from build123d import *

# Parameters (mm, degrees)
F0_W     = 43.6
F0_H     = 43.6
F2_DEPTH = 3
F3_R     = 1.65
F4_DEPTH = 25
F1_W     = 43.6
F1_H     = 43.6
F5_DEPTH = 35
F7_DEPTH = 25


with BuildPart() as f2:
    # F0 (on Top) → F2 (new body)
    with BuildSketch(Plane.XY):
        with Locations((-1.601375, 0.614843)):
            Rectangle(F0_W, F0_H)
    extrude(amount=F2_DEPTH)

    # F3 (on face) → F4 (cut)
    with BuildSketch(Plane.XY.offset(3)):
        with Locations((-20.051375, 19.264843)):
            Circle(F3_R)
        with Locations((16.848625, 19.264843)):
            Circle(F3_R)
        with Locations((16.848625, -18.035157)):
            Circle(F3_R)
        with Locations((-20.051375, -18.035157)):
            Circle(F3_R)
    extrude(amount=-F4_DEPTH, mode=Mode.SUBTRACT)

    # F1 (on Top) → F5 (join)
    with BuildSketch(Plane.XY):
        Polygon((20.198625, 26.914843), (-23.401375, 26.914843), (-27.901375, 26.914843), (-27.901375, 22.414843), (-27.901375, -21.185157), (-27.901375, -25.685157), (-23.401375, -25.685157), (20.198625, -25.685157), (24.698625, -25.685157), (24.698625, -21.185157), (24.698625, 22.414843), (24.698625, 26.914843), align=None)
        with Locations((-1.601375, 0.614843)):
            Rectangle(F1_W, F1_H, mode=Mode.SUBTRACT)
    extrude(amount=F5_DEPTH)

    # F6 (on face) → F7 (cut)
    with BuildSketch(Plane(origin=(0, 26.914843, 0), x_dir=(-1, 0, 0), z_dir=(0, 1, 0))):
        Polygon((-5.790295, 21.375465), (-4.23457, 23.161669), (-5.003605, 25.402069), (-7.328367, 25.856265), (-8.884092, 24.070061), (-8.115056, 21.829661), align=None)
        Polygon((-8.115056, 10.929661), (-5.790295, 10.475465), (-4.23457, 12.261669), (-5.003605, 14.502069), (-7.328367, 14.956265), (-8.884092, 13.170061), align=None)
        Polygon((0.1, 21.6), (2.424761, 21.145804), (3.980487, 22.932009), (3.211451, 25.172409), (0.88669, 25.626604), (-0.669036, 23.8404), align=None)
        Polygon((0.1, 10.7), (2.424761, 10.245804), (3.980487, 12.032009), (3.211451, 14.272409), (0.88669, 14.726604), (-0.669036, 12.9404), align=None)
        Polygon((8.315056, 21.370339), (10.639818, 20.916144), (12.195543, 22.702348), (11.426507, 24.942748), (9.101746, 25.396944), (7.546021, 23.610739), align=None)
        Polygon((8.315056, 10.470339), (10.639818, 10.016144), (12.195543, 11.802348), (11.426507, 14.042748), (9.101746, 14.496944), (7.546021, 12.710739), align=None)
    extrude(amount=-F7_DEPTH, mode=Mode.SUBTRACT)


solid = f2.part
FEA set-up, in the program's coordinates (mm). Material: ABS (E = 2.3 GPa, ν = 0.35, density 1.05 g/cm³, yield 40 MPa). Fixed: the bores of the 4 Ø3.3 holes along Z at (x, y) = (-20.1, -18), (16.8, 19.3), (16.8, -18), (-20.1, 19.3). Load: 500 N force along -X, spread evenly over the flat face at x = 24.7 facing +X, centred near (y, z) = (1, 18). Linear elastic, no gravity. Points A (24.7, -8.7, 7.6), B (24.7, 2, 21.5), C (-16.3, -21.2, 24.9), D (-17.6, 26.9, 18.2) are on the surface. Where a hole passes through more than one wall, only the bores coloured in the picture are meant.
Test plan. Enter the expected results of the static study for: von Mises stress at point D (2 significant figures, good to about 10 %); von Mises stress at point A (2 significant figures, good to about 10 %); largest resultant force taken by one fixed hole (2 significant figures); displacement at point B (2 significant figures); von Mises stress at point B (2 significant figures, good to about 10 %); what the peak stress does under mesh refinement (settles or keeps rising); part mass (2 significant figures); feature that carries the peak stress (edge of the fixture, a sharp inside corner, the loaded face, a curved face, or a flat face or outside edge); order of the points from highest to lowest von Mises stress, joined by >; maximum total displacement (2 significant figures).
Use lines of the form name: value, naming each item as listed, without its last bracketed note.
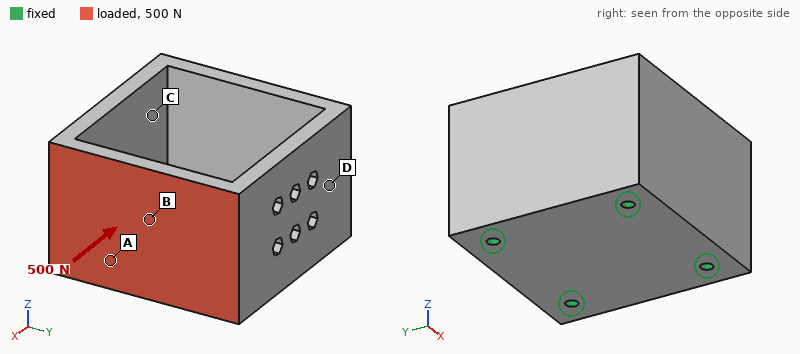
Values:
von Mises stress at point D: 1.9 MPa
von Mises stress at point A: 3.9 MPa
largest resultant force taken by one fixed hole: 180 N
displacement at point B: 0.33 mm
von Mises stress at point B: 6.7 MPa
what the peak stress does under mesh refinement: keeps rising
part mass: 37 g
feature that carries the peak stress: edge of the fixture
order of the points from highest to lowest von Mises stress, joined by >: B > A > D > C
maximum total displacement: 0.52 mm
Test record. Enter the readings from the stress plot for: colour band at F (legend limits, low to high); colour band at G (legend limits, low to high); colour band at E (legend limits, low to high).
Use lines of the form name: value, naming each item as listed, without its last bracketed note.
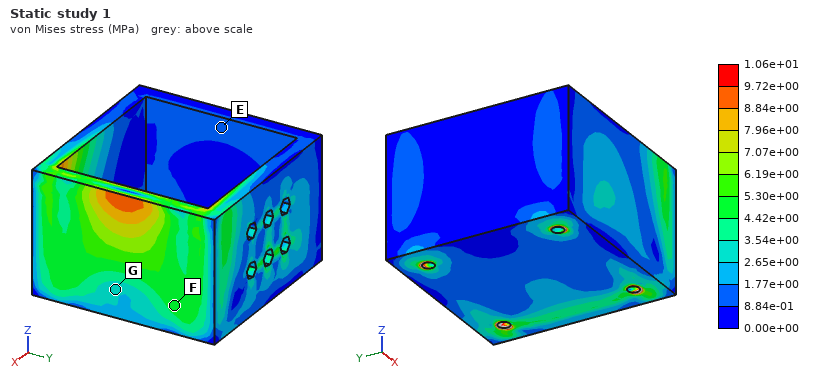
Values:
colour band at F: 4.42e+00 to 5.30e+00 MPa
colour band at G: 2.65e+00 to 3.54e+00 MPa
colour band at E: 8.84e-01 to 1.77e+00 MPa
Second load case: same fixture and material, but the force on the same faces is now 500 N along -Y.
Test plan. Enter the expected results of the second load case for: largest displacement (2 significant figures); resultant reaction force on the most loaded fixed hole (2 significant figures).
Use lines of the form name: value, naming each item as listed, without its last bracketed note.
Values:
largest displacement: 0.18 mm
resultant reaction force on the most loaded fixed hole: 320 N
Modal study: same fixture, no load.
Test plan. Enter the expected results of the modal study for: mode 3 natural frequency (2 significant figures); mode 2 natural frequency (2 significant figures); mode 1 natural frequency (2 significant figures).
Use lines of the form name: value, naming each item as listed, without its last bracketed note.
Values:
mode 3 natural frequency: 2000 Hz
mode 2 natural frequency: 2000 Hz
mode 1 natural frequency: 1900 Hz
